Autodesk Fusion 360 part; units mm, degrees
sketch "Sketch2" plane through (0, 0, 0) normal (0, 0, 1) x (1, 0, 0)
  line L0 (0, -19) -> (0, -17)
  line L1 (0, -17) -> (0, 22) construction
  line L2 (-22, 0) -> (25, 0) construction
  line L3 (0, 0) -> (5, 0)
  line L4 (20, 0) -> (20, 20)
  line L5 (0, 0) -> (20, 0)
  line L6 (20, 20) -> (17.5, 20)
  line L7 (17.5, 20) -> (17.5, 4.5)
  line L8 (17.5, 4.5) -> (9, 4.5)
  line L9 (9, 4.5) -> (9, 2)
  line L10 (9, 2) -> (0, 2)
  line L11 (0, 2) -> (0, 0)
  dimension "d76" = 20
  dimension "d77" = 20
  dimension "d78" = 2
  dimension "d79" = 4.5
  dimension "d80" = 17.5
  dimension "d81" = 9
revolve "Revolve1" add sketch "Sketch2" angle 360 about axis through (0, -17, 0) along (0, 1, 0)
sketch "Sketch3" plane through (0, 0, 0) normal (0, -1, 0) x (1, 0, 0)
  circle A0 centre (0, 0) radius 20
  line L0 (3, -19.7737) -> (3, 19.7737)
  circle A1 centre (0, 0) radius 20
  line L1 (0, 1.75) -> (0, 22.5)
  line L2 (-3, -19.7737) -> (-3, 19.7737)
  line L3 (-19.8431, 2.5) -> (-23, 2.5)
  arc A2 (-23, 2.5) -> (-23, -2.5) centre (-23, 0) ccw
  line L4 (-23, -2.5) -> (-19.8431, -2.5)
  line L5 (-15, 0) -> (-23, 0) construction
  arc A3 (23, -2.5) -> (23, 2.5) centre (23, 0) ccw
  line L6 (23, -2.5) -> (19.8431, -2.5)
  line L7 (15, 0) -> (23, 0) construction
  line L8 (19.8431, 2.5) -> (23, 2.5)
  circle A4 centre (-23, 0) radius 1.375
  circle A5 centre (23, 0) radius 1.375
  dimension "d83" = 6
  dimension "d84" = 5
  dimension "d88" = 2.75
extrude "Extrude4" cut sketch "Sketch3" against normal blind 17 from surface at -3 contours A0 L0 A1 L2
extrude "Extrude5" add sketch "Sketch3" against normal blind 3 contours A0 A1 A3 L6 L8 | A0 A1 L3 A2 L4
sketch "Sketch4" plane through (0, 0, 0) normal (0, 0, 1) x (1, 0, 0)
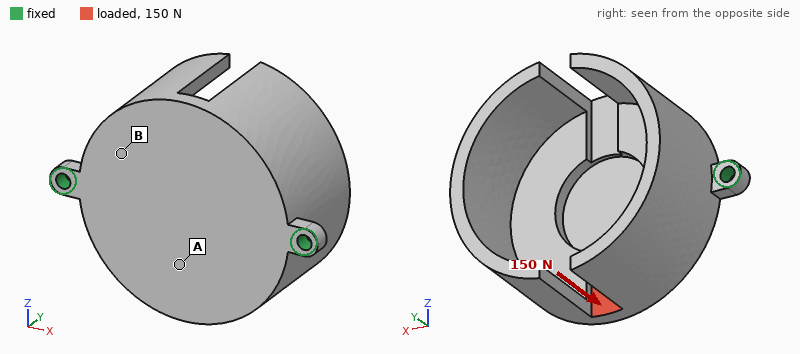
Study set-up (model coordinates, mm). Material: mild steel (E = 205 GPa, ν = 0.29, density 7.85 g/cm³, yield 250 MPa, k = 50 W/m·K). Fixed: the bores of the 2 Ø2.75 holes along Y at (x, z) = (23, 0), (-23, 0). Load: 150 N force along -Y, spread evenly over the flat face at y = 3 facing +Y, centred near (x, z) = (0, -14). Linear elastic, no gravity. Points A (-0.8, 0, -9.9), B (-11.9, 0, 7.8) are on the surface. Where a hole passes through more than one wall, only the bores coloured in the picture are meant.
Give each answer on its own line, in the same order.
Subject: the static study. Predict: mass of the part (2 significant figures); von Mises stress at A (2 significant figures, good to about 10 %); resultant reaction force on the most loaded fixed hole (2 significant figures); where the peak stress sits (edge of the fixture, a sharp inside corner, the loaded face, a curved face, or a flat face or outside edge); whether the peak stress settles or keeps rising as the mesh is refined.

71 g
28 MPa
82 N
edge of the fixture
keeps rising
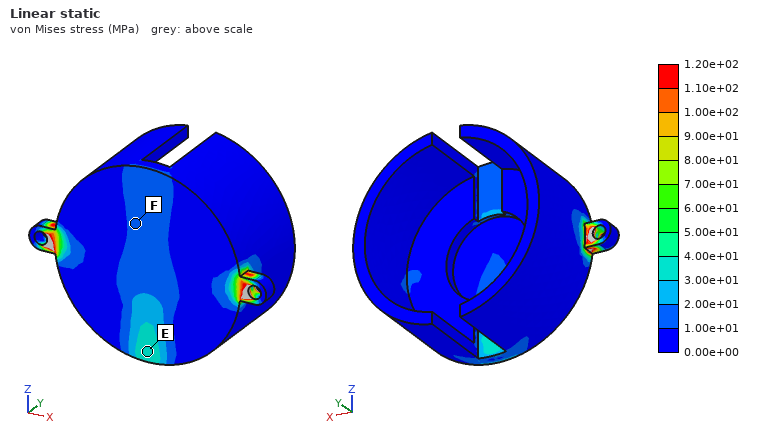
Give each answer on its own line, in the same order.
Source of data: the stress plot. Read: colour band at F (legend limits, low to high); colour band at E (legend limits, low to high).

1.00e+01 to 2.00e+01 MPa
3.00e+01 to 4.00e+01 MPa
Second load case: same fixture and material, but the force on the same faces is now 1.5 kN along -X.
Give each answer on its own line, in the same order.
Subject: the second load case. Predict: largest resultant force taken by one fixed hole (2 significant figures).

910 N
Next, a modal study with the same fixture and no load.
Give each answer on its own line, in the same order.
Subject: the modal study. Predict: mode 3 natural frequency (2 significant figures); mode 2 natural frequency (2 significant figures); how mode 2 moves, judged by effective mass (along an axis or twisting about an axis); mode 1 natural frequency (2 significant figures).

5600 Hz
3300 Hz
along Y
1700 Hz
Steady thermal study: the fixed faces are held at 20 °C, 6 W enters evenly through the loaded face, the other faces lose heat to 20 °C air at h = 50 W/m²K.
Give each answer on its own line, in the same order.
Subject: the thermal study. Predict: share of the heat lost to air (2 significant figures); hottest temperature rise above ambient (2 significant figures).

52 %
25 K
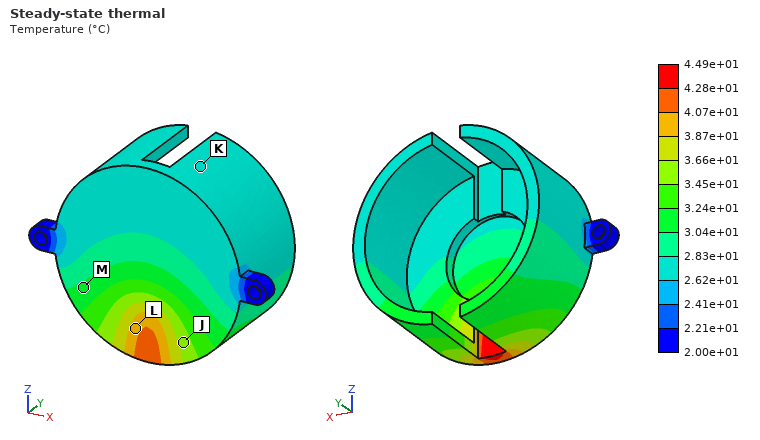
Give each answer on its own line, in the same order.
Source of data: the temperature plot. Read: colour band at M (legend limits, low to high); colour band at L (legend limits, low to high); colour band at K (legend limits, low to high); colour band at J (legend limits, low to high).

3.04e+01 to 3.24e+01 °C
3.87e+01 to 4.07e+01 °C
2.62e+01 to 2.83e+01 °C
3.45e+01 to 3.66e+01 °C
